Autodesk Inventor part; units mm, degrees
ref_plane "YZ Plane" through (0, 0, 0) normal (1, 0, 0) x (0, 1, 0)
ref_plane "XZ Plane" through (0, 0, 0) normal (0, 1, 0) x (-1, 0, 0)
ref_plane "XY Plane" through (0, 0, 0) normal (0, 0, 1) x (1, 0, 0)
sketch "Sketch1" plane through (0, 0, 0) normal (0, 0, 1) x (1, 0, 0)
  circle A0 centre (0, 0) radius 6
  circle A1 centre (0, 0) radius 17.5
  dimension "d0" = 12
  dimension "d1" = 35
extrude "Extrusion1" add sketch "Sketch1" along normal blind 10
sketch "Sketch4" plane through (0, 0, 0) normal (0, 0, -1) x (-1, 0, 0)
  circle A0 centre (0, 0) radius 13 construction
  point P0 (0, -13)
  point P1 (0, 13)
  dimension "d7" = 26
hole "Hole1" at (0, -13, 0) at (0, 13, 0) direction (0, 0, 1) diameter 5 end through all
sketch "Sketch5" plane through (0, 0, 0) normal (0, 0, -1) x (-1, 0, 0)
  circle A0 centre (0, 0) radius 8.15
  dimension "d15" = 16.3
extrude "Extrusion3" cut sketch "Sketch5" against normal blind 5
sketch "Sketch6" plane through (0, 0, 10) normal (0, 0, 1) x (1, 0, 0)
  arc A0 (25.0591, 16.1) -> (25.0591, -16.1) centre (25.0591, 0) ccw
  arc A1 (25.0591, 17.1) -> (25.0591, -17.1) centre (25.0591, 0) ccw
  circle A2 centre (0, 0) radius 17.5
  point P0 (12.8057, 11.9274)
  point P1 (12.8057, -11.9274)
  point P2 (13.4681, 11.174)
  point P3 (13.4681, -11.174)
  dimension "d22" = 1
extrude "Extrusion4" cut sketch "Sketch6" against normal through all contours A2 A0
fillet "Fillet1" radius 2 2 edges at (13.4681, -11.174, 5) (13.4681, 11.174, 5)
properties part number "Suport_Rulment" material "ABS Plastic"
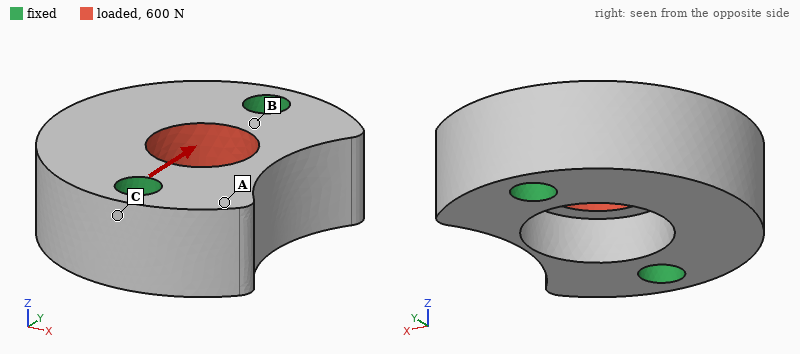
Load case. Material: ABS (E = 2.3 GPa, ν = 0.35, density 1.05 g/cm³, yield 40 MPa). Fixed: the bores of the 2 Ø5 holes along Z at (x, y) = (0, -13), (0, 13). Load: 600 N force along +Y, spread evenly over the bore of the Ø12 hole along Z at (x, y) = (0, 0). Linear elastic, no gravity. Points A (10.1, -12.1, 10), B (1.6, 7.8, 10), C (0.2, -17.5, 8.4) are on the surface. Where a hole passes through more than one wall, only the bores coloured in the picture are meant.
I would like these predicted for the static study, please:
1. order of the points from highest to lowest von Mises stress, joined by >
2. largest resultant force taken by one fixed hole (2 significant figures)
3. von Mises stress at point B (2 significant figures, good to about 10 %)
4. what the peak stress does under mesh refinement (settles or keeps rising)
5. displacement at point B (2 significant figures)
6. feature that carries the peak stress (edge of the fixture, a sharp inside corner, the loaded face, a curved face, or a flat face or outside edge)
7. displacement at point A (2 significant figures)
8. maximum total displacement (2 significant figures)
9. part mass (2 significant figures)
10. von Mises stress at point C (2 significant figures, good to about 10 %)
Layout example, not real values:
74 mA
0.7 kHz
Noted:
B > C > A
300 N
5.1 MPa
keeps rising
8.8 µm
edge of the fixture
16 µm
25 µm
6.6 g
1.8 MPa
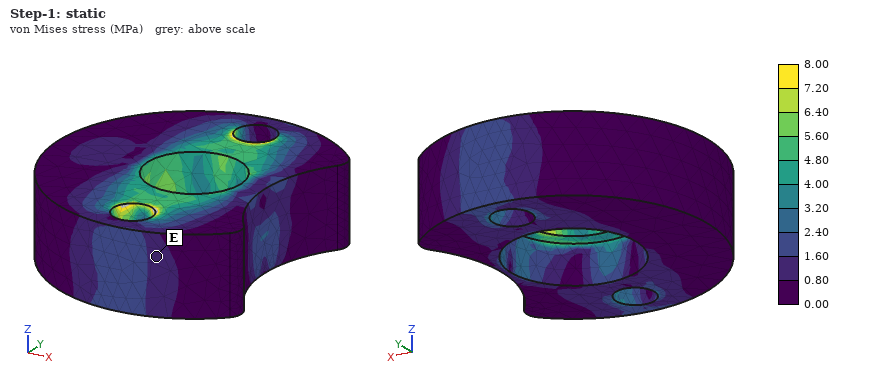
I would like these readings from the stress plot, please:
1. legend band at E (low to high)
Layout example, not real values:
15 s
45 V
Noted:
0.80 to 1.60 MPa
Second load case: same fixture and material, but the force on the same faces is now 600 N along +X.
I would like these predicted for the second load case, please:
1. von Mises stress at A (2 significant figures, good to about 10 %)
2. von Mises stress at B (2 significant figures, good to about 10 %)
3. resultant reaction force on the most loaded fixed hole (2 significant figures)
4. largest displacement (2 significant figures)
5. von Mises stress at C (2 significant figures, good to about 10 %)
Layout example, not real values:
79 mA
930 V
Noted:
1.0 MPa
6.0 MPa
300 N
63 µm
1.1 MPa
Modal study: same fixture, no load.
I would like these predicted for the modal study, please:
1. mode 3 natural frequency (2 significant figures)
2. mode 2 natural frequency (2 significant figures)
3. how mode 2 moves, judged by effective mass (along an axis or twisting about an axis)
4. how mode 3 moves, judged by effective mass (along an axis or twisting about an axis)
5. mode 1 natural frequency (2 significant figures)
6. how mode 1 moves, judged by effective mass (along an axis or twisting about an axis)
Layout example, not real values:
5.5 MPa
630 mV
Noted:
12 kHz
12 kHz
along Y
along Z
6600 Hz
along Z
